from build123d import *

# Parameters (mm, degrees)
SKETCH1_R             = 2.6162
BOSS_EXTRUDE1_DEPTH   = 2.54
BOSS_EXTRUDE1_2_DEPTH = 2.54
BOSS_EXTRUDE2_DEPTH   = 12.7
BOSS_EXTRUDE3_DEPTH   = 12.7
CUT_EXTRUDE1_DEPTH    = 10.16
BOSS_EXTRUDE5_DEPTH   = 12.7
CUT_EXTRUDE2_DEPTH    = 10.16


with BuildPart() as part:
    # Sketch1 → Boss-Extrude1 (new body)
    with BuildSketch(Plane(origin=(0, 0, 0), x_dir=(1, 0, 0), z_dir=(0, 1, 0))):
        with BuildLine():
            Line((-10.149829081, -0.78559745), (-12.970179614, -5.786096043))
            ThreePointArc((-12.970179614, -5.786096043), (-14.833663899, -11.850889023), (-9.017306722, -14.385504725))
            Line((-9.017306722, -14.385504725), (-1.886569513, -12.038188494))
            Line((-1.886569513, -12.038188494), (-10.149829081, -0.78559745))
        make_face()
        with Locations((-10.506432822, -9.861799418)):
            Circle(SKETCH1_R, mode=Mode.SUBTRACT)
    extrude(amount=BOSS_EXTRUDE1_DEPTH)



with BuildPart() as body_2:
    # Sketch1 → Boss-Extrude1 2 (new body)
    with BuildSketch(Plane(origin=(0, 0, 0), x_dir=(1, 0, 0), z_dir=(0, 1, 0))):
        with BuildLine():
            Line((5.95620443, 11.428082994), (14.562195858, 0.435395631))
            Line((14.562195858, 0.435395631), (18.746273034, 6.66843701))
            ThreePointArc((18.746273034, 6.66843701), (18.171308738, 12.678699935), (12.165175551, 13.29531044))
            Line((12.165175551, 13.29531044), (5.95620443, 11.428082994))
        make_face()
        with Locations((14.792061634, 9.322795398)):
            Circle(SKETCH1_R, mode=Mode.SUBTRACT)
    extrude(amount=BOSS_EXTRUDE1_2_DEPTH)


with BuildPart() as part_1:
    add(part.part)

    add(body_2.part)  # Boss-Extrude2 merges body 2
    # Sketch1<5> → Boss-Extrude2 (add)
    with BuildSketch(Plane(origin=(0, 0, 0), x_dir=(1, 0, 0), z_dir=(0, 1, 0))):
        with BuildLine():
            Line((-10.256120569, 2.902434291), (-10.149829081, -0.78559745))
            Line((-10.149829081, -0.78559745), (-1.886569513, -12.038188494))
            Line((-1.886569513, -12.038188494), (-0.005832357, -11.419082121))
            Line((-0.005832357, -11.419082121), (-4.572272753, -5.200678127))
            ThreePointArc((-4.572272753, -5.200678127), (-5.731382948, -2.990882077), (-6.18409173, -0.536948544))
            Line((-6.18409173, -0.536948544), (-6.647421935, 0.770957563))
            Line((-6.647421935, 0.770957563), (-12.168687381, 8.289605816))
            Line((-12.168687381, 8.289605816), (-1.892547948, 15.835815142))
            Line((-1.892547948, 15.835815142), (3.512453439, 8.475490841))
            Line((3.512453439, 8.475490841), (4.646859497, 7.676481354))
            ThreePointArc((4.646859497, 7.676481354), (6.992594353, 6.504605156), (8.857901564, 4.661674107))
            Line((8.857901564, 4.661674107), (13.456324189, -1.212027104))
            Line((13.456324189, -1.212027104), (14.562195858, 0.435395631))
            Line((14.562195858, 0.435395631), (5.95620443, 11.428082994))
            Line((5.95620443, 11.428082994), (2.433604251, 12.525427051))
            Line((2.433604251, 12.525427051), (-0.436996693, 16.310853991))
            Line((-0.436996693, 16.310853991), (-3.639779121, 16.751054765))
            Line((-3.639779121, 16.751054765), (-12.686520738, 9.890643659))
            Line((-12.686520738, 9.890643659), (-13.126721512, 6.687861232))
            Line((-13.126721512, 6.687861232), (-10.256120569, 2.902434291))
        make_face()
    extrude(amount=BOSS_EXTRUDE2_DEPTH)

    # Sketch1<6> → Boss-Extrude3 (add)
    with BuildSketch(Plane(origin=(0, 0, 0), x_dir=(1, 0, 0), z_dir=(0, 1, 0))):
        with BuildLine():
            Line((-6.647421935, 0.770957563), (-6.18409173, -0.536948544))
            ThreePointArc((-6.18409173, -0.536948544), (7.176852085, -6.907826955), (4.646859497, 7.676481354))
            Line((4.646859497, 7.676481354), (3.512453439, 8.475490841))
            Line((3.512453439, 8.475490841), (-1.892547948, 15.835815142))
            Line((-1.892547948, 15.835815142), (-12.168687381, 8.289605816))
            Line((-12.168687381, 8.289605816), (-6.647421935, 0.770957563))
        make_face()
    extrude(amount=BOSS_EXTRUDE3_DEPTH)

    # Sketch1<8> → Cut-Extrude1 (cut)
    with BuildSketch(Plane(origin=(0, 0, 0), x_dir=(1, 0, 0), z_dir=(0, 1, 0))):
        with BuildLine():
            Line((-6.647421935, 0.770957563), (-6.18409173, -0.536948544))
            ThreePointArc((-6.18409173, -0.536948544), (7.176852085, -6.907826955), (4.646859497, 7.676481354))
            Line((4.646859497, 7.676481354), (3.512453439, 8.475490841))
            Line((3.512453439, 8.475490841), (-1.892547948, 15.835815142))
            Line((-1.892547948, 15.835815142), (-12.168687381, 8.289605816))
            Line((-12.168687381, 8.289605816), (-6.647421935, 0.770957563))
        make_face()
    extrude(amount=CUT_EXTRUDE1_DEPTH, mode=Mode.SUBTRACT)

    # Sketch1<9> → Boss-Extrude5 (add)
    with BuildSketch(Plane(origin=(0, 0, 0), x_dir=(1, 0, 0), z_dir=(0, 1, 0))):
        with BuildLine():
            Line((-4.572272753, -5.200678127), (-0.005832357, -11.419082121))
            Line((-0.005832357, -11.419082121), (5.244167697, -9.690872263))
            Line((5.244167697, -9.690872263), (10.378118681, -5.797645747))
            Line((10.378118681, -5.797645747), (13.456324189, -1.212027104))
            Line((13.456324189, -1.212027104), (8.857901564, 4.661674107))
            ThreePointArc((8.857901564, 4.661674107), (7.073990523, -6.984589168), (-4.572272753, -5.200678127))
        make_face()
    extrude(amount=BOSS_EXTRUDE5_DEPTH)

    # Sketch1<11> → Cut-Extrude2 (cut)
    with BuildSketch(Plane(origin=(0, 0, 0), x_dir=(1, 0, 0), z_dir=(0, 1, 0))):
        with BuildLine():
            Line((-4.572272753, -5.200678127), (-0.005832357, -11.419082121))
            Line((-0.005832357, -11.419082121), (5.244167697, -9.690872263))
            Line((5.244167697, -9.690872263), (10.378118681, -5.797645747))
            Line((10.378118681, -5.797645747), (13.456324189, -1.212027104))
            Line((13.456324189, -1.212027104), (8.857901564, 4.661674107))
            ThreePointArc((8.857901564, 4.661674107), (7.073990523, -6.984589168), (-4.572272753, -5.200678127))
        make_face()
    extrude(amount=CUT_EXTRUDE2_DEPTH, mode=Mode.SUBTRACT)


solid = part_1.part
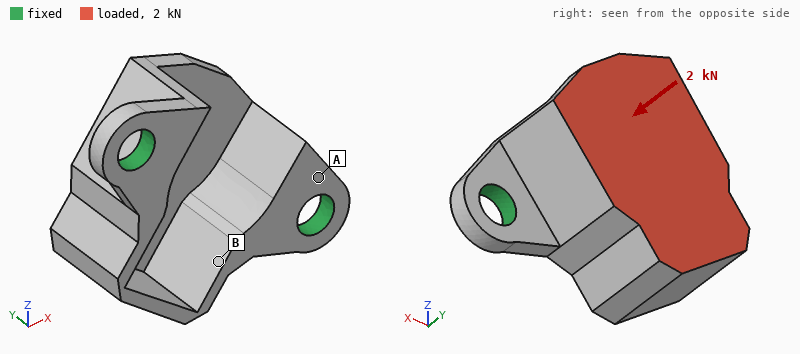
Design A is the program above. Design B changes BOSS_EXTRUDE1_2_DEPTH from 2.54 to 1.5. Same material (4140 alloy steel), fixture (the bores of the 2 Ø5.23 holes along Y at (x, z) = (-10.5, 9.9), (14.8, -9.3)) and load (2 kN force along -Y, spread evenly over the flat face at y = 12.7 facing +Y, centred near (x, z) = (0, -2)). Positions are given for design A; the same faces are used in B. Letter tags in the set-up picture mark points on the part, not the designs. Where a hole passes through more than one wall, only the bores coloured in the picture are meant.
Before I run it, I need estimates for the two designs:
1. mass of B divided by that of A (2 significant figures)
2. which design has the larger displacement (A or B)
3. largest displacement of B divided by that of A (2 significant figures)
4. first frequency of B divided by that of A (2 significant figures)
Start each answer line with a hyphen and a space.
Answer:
- 0.97
- B
- 1.6
- 0.79
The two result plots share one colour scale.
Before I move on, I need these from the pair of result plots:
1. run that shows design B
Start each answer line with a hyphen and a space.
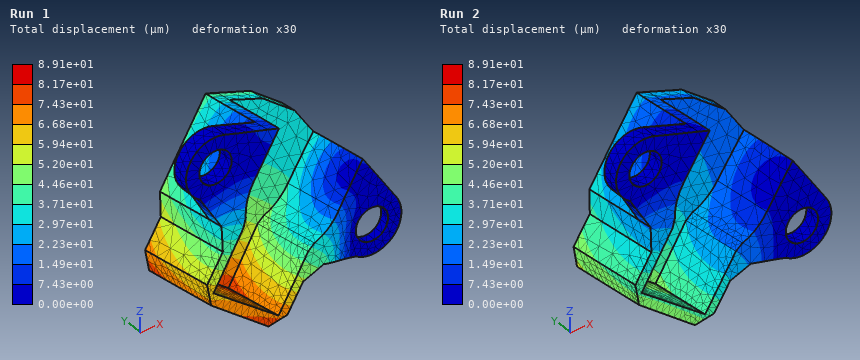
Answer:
- Run 1
